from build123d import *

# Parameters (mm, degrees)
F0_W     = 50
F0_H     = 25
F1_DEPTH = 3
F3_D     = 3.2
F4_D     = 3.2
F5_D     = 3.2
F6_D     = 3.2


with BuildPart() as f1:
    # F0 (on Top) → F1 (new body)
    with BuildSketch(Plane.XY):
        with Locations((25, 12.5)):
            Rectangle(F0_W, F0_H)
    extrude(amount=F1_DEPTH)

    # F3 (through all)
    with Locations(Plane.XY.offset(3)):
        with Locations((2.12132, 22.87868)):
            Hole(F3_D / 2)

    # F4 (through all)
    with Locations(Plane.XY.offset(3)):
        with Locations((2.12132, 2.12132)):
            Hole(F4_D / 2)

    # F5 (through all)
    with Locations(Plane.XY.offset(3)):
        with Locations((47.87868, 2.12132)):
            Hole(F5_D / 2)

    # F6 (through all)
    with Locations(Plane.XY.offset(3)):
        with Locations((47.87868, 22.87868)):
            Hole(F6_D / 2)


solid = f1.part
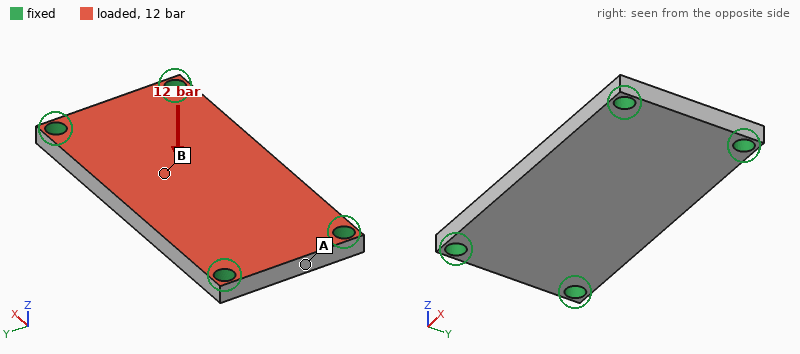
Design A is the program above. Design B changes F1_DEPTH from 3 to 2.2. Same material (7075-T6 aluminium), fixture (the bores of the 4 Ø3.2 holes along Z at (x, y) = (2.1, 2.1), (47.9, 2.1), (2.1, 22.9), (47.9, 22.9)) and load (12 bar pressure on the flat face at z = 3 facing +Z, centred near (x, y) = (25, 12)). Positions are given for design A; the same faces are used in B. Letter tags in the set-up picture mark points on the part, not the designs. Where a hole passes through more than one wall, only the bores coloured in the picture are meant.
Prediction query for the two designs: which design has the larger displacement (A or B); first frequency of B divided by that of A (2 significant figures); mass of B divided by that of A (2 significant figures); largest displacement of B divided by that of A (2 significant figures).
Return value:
B
0.76
0.73
2.4
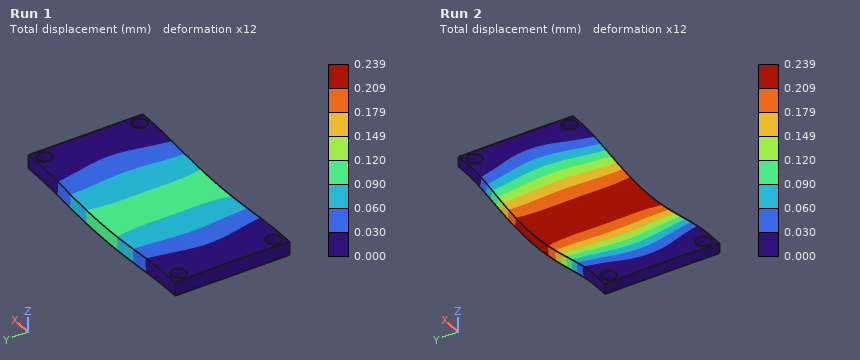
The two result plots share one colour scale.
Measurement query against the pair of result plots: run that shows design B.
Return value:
Run 2
